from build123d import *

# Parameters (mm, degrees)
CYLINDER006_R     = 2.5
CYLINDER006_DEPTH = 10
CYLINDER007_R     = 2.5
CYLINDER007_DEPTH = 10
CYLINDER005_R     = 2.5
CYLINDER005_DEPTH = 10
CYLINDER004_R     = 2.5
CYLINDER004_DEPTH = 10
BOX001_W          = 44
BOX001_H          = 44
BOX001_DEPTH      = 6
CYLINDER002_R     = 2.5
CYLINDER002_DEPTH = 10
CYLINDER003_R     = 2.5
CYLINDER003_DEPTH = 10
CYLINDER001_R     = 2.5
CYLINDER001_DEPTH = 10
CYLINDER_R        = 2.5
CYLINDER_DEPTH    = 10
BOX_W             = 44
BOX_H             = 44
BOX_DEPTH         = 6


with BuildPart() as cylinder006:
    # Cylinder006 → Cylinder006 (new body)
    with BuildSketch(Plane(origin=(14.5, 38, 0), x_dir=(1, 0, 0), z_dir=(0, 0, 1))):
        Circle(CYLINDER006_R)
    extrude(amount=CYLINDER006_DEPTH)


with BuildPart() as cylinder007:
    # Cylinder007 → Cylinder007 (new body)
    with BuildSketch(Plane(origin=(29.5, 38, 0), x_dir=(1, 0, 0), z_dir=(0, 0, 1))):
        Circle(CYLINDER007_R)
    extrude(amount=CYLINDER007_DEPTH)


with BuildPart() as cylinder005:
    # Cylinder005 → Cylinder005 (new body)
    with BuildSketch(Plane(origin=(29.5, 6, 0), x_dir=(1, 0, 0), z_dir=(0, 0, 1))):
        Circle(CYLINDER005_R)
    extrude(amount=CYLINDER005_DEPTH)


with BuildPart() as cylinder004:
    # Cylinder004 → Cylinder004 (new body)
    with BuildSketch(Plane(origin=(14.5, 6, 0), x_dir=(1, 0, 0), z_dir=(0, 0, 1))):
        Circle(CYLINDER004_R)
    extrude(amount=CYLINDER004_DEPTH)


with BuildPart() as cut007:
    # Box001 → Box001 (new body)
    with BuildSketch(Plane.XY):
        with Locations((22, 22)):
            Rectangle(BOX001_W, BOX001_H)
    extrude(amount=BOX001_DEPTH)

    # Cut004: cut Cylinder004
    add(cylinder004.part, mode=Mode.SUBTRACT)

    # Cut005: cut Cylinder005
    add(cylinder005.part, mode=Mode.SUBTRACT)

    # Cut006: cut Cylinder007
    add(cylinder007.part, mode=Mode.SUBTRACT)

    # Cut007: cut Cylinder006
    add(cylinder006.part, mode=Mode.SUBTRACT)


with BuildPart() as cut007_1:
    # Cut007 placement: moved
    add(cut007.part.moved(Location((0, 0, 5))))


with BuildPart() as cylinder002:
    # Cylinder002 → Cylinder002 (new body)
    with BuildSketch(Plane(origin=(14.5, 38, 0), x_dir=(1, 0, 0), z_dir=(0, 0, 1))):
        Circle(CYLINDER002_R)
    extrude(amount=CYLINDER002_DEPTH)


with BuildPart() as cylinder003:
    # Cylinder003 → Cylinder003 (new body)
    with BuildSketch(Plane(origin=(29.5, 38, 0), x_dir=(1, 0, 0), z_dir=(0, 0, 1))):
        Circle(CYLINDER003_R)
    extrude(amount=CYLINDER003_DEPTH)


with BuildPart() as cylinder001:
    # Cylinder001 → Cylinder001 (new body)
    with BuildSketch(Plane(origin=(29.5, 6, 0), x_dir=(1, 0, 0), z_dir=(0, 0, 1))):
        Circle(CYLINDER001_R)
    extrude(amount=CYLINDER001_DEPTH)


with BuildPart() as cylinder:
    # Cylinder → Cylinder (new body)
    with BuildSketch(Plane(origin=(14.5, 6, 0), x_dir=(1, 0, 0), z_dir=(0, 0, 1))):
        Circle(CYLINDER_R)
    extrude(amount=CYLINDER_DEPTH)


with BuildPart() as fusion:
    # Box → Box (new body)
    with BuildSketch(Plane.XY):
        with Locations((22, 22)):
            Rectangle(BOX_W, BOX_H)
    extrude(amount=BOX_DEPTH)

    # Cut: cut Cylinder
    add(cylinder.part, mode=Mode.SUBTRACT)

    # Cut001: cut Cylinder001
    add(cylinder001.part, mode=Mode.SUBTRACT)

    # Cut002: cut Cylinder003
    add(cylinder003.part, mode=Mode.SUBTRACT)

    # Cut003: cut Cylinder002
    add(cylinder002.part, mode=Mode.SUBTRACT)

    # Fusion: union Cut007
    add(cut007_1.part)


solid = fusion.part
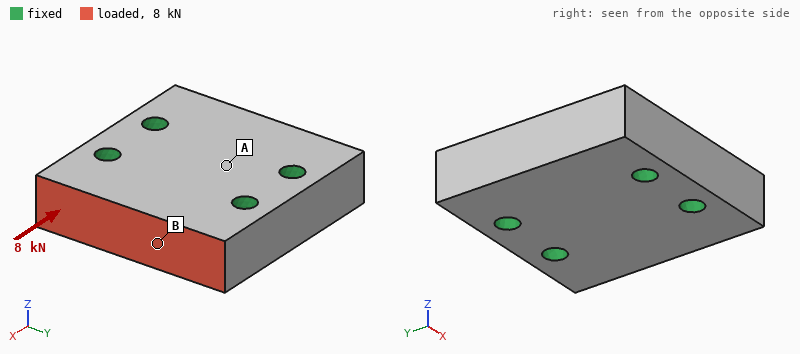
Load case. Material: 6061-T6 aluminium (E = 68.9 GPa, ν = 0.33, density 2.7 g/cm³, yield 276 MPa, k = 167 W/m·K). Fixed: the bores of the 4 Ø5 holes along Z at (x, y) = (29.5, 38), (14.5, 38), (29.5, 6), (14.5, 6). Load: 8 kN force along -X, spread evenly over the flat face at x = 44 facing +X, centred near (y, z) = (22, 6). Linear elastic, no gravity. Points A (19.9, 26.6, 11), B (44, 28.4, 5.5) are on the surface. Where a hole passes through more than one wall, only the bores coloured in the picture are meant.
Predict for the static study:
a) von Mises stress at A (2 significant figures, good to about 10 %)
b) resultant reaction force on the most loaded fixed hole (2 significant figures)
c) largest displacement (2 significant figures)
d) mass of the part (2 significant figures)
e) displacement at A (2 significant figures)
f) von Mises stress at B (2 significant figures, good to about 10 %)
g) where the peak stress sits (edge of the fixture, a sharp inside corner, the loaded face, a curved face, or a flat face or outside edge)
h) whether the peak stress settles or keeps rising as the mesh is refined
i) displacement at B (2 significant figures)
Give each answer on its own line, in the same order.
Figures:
6.3 MPa
3.2 kN
5.4 µm
55 g
1.6 µm
14 MPa
edge of the fixture
keeps rising
4.9 µm
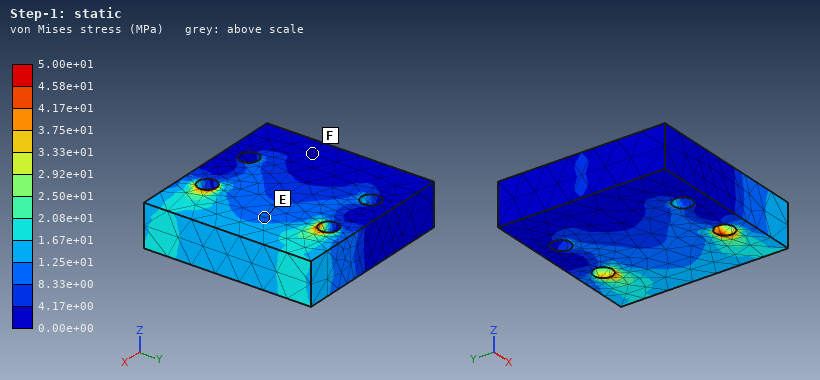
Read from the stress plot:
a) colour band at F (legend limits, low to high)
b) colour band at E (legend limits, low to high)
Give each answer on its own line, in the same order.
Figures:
0.00e+00 to 4.17e+00 MPa
8.33e+00 to 1.25e+01 MPa
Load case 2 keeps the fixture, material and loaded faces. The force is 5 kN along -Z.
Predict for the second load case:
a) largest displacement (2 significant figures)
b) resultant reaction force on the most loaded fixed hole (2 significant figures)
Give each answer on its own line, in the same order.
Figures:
34 µm
2.9 kN
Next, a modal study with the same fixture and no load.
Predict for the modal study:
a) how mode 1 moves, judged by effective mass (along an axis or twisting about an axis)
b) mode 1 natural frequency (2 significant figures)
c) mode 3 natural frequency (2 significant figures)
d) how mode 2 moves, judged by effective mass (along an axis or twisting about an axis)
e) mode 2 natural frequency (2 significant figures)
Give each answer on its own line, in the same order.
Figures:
twisting about Y
25 kHz
38 kHz
along Z
26 kHz
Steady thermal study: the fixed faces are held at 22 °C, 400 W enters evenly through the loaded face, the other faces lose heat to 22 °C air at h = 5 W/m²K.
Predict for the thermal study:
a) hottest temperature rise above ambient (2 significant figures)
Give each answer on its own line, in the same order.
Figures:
84 K
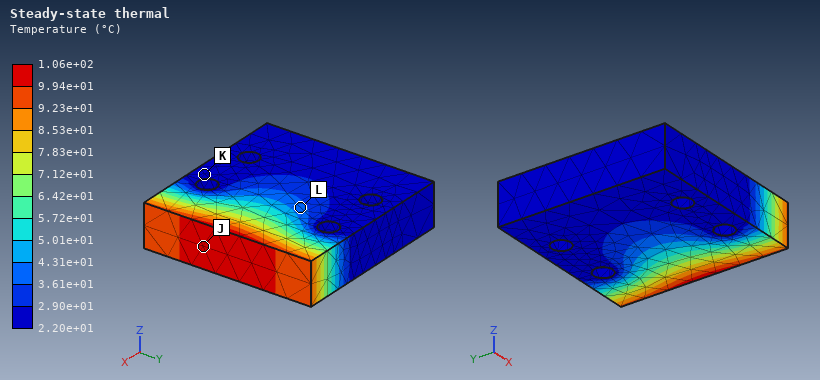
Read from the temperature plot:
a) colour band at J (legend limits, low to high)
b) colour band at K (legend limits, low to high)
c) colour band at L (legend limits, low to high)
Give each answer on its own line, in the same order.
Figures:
9.94e+01 to 1.06e+02 °C
2.20e+01 to 2.90e+01 °C
3.61e+01 to 4.31e+01 °C
